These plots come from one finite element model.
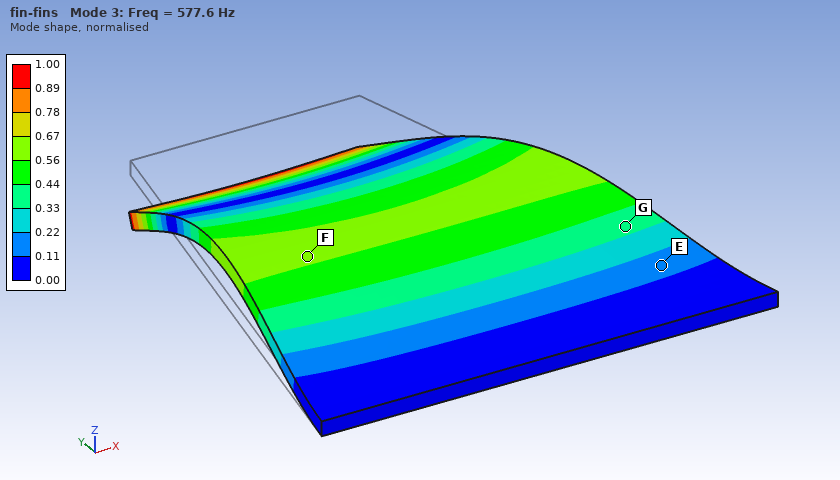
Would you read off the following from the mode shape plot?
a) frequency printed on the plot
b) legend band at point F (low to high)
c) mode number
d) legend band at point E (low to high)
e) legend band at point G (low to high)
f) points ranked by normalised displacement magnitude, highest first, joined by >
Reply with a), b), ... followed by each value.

a) 577.6 Hz
b) 0.56 to 0.67
c) 3
d) 0.11 to 0.22
e) 0.33 to 0.44
f) F > G > E
